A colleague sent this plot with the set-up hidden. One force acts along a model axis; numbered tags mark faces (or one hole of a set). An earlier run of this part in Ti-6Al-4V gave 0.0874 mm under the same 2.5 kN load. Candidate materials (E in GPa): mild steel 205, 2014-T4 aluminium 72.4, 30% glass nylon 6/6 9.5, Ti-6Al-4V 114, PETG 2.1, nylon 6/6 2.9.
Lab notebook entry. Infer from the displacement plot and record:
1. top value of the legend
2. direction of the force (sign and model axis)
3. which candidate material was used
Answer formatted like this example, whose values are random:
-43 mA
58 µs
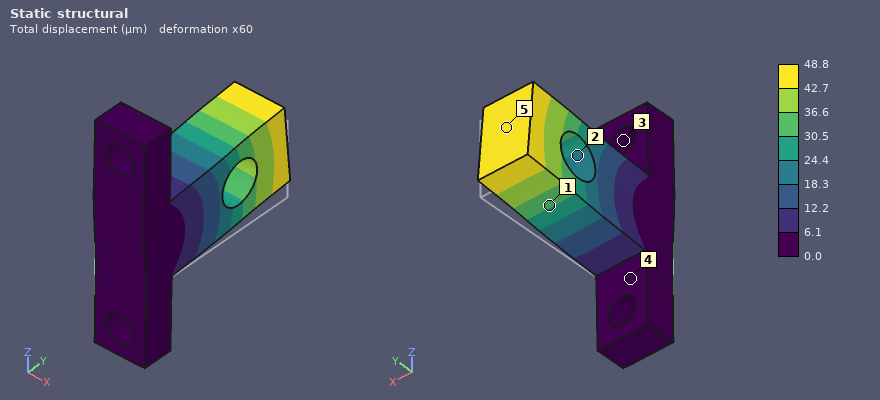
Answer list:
48.8 µm
+Z
mild steel
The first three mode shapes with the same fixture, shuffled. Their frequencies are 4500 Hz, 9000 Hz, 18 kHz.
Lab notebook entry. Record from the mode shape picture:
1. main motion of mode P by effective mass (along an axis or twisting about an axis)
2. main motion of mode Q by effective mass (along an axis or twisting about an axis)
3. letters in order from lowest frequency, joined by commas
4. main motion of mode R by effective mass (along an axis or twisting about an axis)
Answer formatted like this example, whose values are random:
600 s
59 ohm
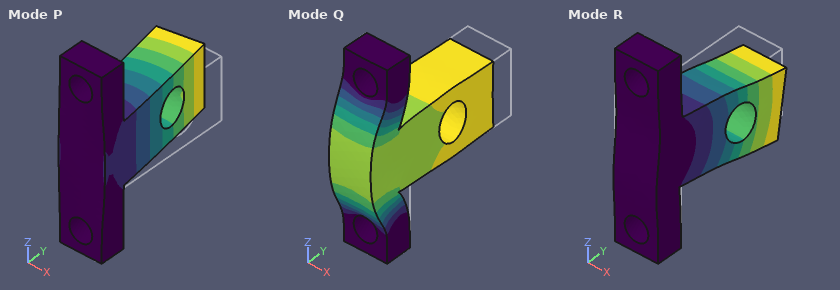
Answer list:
along X
along Y
P, R, Q
along Z
